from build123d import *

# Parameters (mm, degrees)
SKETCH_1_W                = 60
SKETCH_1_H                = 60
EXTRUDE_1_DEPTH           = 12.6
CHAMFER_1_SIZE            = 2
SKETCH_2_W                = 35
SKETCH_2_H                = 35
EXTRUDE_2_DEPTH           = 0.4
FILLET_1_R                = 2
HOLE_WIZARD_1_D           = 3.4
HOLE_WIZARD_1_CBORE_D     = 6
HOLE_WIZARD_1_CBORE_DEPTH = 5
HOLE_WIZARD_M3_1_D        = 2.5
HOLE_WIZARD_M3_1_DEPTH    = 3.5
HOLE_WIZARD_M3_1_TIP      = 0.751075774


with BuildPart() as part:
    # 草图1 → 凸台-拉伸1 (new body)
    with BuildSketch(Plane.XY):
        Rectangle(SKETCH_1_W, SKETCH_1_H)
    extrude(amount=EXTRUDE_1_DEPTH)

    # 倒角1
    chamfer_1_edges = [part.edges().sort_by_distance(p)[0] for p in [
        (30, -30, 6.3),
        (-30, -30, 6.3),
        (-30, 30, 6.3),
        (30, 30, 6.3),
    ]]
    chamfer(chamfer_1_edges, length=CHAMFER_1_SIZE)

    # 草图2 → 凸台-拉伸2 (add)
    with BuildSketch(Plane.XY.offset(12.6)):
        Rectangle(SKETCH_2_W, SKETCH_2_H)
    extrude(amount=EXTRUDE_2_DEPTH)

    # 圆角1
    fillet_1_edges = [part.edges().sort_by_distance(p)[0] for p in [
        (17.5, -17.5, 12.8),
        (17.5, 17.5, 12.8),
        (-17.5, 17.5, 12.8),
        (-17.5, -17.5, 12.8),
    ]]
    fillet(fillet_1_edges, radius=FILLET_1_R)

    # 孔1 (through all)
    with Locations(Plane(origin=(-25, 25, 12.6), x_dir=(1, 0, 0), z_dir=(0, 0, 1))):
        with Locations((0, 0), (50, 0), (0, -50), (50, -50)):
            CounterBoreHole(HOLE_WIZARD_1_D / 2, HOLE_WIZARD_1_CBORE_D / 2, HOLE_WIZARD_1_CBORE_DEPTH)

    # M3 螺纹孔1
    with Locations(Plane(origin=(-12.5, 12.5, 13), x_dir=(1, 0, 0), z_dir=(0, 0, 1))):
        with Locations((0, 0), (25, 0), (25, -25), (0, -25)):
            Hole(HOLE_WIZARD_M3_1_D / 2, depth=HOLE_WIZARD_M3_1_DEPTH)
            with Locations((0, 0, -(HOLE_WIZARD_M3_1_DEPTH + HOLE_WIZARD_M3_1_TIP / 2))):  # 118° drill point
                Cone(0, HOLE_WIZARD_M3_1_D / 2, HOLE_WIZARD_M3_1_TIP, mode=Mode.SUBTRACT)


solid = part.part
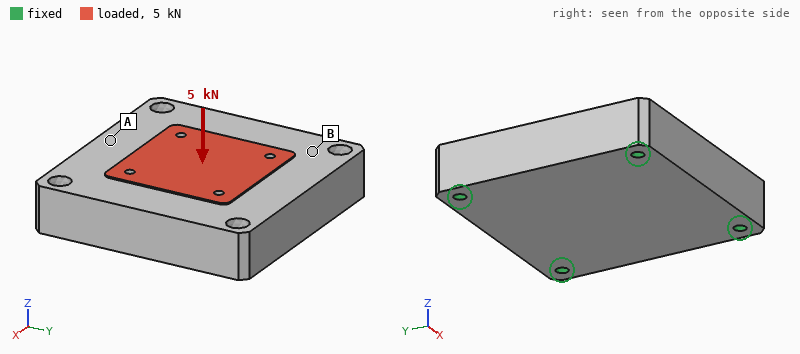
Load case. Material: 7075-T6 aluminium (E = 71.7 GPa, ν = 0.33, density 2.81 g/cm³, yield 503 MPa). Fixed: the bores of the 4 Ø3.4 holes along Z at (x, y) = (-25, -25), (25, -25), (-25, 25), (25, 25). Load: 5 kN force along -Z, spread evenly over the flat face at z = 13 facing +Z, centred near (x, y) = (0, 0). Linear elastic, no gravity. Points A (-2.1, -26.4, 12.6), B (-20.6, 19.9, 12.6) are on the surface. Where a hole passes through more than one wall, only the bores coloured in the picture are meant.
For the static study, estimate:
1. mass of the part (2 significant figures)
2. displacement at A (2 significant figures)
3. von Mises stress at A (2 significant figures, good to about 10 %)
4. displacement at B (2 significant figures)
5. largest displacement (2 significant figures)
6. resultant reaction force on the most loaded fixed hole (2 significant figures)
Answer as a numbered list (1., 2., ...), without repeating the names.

1. 130 g
2. 9.3 µm
3. 16 MPa
4. 6.6 µm
5. 18 µm
6. 1.5 kN
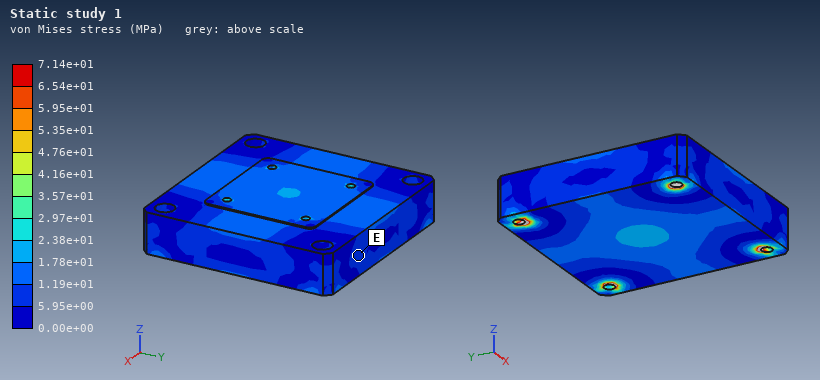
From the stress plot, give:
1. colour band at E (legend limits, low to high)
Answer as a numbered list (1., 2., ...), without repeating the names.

1. 5.95e+00 to 1.19e+01 MPa
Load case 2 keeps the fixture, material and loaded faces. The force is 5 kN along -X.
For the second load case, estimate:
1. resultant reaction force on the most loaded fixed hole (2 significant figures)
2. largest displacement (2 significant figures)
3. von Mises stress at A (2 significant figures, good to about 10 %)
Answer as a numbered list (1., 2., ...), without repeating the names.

1. 1.4 kN
2. 5.4 µm
3. 4.0 MPa
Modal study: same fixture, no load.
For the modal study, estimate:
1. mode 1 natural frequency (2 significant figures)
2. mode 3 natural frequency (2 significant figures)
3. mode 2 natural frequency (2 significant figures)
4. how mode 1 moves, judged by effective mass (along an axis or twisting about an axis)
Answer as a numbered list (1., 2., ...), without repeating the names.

1. 11 kHz
2. 17 kHz
3. 17 kHz
4. along Z
